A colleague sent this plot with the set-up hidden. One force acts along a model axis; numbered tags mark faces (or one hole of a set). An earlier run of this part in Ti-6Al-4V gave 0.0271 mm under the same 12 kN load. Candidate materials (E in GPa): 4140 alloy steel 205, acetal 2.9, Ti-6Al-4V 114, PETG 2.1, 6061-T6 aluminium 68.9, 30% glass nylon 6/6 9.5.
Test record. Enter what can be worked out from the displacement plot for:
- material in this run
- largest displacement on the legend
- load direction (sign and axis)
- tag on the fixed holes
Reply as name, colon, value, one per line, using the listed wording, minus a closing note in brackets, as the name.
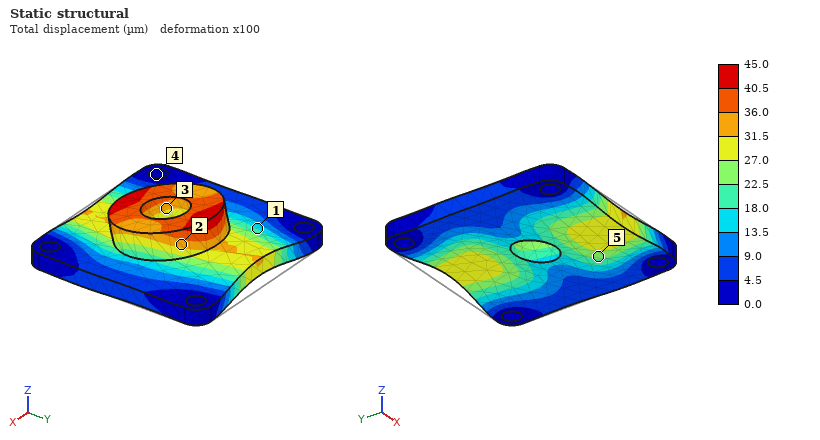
material in this run: 6061-T6 aluminium
largest displacement on the legend: 45.0 µm
load direction: -Y
tag on the fixed holes: 4
